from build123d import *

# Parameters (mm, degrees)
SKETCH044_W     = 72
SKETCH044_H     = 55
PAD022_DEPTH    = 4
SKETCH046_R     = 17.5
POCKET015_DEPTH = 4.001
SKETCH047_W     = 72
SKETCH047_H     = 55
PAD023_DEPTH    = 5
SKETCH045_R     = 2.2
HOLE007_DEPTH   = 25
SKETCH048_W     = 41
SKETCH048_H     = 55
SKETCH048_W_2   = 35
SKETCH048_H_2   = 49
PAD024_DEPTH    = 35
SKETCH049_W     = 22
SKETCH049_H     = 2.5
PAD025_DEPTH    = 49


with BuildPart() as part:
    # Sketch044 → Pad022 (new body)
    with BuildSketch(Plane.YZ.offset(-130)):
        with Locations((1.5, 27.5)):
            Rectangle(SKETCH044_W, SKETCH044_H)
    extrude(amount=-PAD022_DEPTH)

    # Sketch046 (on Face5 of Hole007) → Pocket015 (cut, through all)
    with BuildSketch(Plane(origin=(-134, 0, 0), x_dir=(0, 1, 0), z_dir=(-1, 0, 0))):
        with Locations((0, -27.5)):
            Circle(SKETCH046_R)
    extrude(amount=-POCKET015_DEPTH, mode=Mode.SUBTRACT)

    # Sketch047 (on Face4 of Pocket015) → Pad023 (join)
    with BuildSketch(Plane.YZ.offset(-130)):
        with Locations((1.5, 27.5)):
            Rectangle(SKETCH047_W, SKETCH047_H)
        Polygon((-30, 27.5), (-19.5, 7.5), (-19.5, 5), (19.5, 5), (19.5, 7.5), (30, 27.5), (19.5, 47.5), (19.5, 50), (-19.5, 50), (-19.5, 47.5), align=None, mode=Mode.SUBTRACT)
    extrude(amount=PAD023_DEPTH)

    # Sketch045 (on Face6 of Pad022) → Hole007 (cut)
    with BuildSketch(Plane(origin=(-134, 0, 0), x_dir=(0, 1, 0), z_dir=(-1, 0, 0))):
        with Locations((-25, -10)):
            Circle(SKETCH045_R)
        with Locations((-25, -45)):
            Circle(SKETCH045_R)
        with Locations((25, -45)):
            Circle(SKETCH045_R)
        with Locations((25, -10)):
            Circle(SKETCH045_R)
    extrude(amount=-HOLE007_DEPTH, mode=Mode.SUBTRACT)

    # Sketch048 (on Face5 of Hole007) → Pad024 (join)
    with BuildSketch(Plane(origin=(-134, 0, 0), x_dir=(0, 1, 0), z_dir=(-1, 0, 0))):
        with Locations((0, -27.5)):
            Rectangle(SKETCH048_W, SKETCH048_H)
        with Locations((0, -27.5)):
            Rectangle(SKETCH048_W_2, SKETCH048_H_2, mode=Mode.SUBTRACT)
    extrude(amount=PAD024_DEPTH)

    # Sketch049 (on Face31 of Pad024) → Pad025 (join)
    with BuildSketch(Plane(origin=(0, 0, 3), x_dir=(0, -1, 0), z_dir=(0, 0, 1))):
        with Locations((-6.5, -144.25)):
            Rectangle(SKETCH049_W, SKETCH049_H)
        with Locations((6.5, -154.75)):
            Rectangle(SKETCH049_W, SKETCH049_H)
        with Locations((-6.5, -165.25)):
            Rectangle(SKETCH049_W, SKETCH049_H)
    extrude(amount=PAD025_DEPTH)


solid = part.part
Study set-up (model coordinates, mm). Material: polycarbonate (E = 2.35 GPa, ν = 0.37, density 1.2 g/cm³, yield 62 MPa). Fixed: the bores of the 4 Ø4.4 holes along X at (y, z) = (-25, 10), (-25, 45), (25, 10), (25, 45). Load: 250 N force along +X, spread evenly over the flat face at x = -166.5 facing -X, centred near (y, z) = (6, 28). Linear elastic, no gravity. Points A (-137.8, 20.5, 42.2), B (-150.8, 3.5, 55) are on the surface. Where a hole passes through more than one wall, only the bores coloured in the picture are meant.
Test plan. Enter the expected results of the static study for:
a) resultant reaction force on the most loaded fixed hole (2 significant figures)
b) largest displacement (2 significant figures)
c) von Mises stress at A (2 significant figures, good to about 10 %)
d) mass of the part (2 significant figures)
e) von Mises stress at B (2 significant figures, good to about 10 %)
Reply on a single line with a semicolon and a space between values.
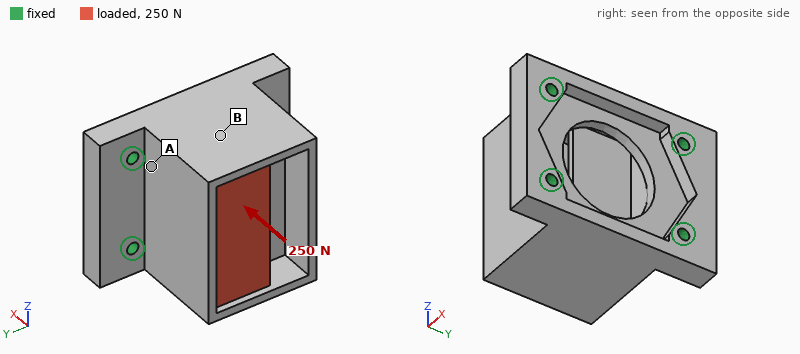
84 N; 1.0 mm; 2.4 MPa; 57 g; 1.3 MPa
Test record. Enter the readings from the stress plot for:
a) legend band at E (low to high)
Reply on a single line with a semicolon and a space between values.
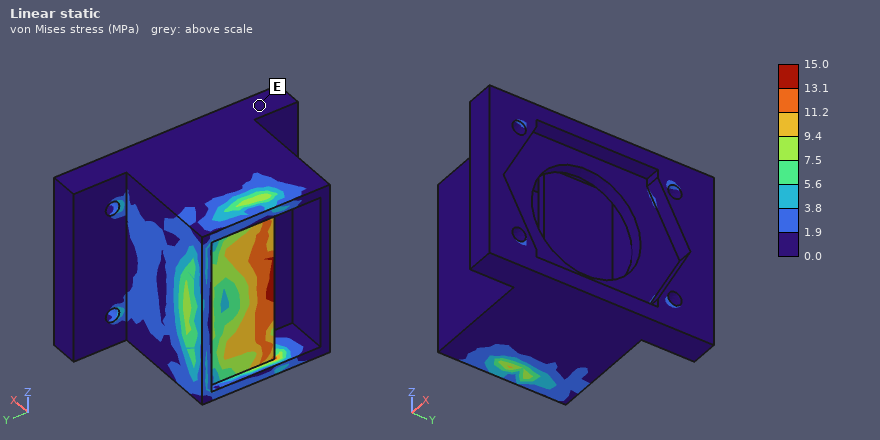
0.0 to 1.9 MPa
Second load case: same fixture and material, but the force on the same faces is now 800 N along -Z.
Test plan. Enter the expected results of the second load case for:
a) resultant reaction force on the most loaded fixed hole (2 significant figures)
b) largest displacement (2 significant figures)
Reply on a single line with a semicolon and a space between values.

540 N; 0.50 mm
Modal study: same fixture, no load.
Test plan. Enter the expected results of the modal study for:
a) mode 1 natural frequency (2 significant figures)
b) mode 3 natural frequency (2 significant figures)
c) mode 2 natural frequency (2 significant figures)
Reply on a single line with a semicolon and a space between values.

1900 Hz; 2000 Hz; 1900 Hz
